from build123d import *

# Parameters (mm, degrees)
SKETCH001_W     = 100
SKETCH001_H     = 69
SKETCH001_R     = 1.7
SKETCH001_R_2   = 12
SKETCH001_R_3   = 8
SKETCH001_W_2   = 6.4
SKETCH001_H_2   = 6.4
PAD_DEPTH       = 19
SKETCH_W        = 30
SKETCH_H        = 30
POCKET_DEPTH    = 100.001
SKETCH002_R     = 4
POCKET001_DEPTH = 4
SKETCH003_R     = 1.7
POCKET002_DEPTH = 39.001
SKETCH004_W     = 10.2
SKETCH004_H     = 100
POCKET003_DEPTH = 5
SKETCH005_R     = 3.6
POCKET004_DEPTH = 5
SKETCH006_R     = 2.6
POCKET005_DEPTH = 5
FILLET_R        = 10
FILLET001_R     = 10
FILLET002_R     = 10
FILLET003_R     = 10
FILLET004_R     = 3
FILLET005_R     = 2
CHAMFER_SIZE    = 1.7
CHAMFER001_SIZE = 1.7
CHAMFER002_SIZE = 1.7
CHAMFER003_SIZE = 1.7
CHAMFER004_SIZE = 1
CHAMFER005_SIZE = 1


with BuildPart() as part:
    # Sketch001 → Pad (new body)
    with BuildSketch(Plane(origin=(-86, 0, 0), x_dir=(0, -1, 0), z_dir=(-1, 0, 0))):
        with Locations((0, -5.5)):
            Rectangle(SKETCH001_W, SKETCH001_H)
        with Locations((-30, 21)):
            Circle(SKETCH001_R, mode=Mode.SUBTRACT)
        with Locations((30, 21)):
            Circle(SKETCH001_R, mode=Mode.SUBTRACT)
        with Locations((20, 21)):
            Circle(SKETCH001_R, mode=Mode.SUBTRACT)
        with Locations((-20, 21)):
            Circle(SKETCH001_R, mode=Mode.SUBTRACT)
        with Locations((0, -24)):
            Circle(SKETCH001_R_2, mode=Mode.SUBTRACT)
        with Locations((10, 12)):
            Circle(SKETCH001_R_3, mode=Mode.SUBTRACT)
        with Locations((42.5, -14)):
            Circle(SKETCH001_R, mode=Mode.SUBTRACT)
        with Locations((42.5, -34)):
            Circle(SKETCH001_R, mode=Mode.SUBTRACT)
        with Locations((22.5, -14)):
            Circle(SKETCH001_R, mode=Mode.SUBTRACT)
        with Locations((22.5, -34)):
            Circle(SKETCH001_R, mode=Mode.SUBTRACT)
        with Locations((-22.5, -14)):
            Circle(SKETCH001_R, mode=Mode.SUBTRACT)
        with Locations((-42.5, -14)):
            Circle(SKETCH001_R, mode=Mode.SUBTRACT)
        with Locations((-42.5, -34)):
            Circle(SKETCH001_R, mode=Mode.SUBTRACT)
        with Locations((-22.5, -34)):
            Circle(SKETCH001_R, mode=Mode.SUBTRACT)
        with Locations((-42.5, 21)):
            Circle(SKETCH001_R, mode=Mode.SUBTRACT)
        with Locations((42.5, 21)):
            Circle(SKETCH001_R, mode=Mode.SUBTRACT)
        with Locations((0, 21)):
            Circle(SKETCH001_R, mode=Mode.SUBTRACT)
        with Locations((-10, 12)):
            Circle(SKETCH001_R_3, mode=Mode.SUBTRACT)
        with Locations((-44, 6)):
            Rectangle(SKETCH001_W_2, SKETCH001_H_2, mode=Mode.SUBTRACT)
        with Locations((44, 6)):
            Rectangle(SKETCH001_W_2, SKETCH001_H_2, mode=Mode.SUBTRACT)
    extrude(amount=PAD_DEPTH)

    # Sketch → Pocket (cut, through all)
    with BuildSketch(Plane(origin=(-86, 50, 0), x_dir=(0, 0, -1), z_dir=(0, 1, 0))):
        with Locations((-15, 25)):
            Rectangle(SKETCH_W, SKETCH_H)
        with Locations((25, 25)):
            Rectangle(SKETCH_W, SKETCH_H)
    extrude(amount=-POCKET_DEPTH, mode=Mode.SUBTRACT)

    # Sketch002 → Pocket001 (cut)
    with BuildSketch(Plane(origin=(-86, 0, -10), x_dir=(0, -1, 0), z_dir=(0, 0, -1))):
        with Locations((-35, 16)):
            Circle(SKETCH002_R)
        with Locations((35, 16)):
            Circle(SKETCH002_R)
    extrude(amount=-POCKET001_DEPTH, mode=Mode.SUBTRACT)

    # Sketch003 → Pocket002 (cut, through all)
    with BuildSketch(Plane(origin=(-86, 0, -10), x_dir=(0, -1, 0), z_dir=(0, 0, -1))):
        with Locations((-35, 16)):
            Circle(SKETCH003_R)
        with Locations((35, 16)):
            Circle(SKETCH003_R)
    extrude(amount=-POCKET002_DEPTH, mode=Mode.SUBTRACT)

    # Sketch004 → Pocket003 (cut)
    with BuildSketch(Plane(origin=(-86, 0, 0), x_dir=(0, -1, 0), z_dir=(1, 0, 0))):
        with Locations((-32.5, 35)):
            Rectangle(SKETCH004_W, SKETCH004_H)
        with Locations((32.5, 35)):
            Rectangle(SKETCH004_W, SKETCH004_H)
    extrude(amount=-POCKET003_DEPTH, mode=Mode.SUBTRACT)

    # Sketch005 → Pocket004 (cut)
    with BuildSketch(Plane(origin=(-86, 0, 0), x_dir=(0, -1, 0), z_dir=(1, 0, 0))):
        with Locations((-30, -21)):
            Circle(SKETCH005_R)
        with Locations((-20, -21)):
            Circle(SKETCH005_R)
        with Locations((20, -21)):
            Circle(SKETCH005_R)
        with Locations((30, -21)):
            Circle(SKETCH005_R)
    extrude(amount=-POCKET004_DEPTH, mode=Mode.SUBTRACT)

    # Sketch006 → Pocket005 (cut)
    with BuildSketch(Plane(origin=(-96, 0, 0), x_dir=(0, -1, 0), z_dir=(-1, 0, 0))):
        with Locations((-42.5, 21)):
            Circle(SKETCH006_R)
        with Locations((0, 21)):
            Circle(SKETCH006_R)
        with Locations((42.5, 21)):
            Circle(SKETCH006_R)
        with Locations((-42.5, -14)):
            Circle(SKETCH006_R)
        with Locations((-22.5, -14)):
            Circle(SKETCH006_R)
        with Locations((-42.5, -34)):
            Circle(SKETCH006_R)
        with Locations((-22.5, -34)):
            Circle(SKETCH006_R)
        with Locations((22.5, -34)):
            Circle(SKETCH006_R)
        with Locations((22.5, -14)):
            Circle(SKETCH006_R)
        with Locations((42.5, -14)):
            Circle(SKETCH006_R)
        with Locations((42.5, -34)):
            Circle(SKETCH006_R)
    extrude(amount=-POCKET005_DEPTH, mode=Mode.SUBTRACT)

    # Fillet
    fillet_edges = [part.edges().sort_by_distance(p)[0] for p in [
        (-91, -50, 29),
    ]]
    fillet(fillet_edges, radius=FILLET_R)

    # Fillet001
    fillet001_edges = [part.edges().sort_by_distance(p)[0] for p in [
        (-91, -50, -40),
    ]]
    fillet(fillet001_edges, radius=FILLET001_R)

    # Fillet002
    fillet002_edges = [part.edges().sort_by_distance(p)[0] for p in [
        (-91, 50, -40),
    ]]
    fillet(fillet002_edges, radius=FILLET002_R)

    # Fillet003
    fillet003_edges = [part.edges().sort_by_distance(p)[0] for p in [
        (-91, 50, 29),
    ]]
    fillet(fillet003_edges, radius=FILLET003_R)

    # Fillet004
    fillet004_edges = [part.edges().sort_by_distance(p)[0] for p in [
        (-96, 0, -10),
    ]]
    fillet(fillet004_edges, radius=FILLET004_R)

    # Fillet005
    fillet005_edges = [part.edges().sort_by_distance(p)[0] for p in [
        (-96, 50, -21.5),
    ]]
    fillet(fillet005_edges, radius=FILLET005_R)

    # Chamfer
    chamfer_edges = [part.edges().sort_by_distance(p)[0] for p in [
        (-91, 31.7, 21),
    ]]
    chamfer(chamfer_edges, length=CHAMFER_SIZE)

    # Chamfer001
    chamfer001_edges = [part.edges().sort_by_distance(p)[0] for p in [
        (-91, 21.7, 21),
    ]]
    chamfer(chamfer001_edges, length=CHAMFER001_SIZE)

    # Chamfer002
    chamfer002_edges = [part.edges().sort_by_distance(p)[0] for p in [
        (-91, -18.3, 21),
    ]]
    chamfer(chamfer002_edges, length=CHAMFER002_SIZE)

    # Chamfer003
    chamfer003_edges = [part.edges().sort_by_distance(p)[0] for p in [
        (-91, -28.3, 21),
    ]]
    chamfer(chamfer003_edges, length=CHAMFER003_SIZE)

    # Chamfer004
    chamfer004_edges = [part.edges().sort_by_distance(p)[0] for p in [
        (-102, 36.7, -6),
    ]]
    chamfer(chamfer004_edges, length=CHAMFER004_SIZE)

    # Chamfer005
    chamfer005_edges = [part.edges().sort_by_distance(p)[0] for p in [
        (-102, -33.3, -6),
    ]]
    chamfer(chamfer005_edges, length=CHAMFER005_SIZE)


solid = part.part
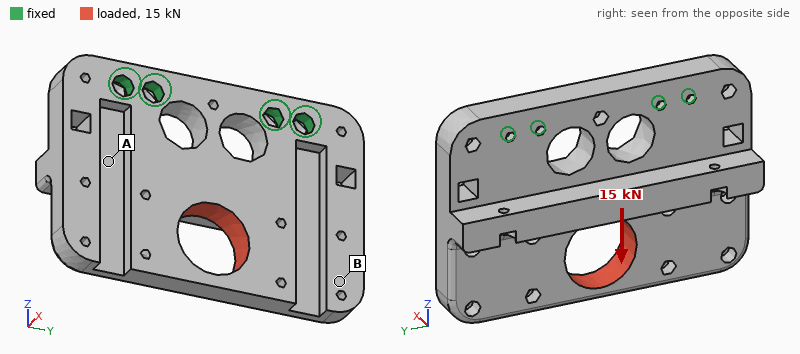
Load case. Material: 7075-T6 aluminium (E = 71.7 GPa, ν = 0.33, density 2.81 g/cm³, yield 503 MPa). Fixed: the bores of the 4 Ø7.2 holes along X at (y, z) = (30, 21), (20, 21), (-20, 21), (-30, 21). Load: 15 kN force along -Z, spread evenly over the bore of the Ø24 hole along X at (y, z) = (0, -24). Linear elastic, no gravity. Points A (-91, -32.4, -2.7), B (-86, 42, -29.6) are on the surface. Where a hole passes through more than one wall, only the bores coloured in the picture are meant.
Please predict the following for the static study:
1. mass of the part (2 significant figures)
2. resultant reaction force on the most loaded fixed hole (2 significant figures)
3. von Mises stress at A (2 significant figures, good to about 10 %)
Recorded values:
170 g
4.0 kN
22 MPa
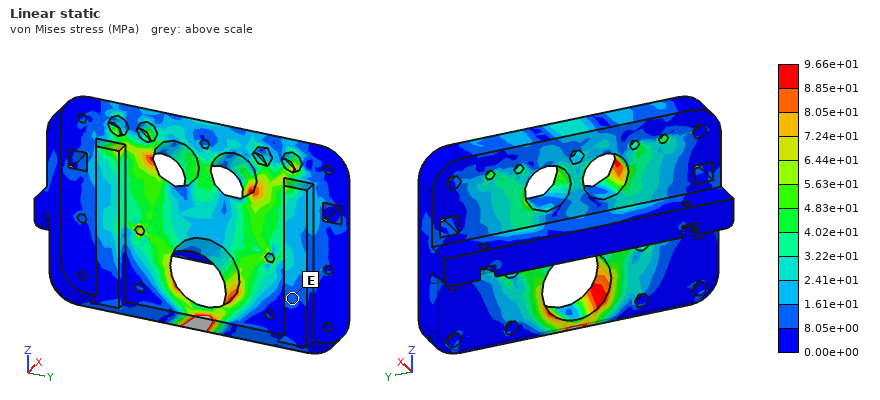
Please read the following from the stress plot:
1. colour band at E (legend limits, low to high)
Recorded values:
8.05e+00 to 1.61e+01 MPa
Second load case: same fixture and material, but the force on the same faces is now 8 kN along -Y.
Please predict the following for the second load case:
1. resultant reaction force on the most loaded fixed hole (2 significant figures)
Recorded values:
6.0 kN
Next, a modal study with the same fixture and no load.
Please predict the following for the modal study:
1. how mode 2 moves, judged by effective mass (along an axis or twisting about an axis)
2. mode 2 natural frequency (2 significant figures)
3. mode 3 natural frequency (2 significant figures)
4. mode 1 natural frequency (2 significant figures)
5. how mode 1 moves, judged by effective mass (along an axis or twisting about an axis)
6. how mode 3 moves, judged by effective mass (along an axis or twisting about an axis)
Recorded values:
twisting about Z
3000 Hz
6100 Hz
1700 Hz
along X
along Y
